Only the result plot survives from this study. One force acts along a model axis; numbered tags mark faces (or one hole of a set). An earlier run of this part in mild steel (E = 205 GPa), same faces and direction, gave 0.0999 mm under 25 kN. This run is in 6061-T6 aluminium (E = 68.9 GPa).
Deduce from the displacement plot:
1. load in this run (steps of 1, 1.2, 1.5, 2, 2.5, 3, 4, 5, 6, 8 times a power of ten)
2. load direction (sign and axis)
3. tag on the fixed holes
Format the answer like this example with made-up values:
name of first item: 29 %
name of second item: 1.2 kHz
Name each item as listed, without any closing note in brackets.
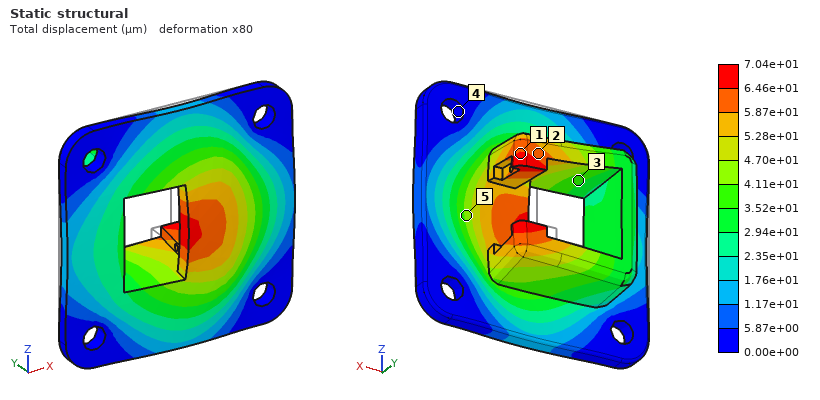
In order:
load in this run: 6 kN
load direction: -Y
tag on the fixed holes: 4
